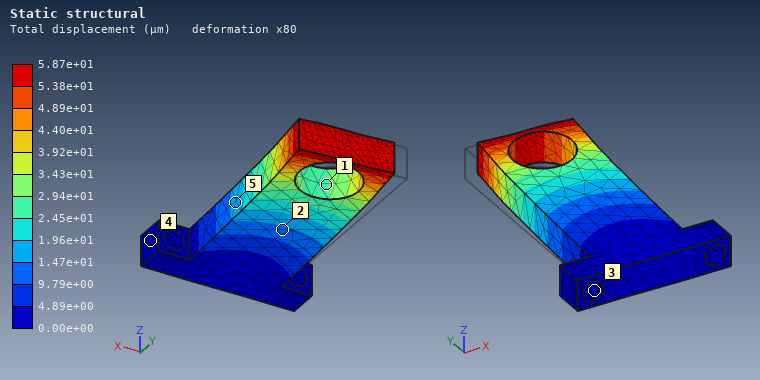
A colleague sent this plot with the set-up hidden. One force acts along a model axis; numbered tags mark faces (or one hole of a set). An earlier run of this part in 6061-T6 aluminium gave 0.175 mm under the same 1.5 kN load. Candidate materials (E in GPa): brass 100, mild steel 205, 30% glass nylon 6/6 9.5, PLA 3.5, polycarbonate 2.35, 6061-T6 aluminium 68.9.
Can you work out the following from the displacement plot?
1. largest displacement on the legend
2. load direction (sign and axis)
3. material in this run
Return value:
5.87e+01 µm
+X
mild steel
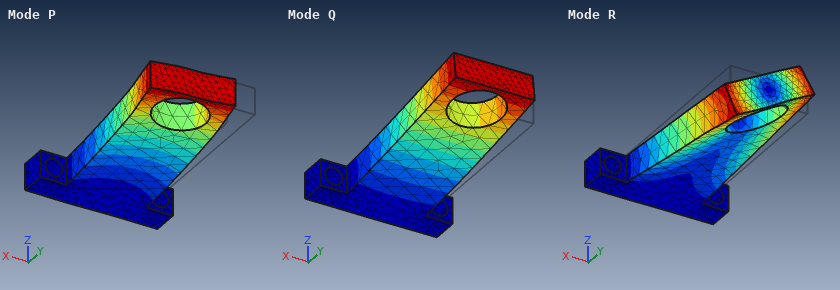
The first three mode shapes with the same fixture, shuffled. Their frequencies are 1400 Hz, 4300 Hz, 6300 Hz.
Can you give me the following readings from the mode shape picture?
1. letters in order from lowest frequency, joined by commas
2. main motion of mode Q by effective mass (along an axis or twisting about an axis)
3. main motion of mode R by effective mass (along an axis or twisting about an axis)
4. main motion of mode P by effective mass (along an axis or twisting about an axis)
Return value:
Q, P, R
along Z
twisting about Y
along X
